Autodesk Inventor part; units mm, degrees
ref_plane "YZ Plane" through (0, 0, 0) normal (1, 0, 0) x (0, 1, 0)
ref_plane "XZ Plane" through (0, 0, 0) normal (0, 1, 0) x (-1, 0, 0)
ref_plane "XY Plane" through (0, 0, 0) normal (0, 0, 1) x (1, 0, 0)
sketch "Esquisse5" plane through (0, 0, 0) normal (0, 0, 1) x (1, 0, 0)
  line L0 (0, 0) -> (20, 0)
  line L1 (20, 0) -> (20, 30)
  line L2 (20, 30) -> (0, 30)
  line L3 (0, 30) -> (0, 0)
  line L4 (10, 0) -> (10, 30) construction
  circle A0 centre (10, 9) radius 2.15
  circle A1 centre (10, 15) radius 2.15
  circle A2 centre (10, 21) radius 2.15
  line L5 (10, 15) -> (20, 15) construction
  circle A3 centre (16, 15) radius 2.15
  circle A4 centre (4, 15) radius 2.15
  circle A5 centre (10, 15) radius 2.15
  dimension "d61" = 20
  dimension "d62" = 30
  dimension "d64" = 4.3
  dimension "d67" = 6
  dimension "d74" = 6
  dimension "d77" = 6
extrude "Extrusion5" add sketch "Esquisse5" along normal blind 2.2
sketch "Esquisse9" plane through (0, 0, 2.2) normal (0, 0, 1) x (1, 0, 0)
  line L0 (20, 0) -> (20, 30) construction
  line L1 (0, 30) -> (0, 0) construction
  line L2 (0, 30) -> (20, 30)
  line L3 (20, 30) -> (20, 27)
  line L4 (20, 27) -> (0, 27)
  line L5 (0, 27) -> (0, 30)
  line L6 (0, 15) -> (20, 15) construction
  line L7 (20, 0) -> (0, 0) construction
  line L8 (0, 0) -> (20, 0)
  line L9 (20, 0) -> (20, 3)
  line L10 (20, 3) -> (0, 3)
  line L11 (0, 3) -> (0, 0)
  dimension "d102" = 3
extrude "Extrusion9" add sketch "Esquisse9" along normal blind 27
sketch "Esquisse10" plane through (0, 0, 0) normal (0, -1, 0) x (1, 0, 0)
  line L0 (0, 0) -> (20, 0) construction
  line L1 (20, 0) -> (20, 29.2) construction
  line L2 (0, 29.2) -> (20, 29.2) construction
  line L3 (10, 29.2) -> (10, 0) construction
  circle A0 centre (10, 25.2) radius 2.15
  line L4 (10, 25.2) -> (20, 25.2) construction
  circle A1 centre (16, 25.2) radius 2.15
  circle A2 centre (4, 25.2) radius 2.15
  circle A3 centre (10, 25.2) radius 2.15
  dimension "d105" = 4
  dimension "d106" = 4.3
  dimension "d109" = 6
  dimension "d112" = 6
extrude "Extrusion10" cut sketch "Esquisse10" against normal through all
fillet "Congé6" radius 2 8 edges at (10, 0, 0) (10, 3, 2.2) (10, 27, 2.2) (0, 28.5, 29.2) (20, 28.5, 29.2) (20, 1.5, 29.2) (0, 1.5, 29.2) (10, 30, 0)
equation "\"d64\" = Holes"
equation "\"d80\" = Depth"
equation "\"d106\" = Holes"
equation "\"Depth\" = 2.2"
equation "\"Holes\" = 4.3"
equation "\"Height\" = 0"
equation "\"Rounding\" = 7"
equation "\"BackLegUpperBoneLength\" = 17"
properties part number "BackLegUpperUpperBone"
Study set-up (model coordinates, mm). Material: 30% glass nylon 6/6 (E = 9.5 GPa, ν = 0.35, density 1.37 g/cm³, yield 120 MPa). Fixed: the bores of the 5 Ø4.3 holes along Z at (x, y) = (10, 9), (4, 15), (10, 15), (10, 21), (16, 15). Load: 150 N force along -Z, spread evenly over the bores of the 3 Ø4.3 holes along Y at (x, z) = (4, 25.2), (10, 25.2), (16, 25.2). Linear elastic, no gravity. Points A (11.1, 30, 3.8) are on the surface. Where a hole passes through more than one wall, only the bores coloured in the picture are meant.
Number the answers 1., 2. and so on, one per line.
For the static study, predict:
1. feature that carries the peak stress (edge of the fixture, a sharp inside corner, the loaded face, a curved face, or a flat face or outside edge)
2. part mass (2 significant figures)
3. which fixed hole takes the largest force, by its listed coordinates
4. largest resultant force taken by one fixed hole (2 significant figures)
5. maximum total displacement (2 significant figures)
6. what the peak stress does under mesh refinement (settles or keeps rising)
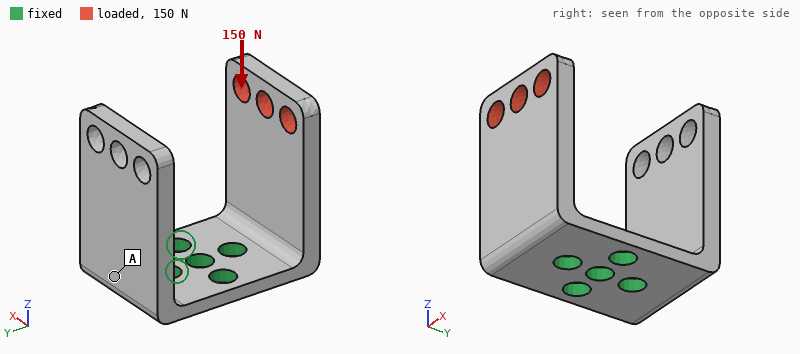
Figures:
1. edge of the fixture
2. 5.7 g
3. (10, 9)
4. 190 N
5. 0.52 mm
6. keeps rising
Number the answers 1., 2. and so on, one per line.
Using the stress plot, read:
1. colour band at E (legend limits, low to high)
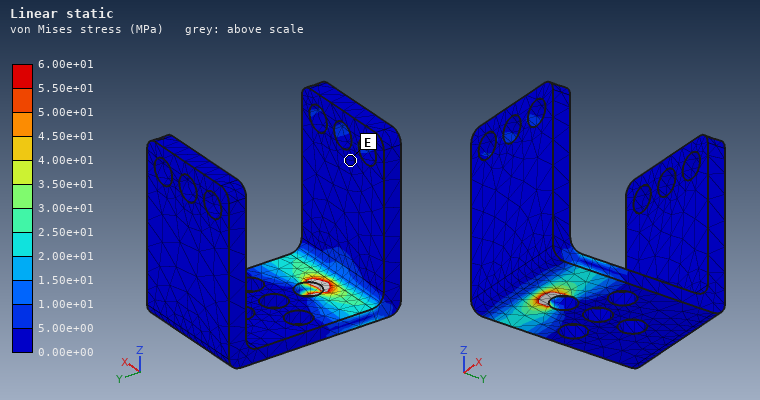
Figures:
1. 0.00e+00 to 5.00e+00 MPa
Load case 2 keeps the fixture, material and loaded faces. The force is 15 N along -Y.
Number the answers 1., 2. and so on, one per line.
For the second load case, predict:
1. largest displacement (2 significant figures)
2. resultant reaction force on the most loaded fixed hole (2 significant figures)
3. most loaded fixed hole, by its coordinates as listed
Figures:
1. 0.46 mm
2. 30 N
3. (10, 9)
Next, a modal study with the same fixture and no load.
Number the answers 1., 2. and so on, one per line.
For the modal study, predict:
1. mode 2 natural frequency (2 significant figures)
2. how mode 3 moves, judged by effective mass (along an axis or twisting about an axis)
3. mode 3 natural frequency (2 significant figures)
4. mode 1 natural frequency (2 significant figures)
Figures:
1. 1100 Hz
2. twisting about Z
3. 1900 Hz
4. 1100 Hz
